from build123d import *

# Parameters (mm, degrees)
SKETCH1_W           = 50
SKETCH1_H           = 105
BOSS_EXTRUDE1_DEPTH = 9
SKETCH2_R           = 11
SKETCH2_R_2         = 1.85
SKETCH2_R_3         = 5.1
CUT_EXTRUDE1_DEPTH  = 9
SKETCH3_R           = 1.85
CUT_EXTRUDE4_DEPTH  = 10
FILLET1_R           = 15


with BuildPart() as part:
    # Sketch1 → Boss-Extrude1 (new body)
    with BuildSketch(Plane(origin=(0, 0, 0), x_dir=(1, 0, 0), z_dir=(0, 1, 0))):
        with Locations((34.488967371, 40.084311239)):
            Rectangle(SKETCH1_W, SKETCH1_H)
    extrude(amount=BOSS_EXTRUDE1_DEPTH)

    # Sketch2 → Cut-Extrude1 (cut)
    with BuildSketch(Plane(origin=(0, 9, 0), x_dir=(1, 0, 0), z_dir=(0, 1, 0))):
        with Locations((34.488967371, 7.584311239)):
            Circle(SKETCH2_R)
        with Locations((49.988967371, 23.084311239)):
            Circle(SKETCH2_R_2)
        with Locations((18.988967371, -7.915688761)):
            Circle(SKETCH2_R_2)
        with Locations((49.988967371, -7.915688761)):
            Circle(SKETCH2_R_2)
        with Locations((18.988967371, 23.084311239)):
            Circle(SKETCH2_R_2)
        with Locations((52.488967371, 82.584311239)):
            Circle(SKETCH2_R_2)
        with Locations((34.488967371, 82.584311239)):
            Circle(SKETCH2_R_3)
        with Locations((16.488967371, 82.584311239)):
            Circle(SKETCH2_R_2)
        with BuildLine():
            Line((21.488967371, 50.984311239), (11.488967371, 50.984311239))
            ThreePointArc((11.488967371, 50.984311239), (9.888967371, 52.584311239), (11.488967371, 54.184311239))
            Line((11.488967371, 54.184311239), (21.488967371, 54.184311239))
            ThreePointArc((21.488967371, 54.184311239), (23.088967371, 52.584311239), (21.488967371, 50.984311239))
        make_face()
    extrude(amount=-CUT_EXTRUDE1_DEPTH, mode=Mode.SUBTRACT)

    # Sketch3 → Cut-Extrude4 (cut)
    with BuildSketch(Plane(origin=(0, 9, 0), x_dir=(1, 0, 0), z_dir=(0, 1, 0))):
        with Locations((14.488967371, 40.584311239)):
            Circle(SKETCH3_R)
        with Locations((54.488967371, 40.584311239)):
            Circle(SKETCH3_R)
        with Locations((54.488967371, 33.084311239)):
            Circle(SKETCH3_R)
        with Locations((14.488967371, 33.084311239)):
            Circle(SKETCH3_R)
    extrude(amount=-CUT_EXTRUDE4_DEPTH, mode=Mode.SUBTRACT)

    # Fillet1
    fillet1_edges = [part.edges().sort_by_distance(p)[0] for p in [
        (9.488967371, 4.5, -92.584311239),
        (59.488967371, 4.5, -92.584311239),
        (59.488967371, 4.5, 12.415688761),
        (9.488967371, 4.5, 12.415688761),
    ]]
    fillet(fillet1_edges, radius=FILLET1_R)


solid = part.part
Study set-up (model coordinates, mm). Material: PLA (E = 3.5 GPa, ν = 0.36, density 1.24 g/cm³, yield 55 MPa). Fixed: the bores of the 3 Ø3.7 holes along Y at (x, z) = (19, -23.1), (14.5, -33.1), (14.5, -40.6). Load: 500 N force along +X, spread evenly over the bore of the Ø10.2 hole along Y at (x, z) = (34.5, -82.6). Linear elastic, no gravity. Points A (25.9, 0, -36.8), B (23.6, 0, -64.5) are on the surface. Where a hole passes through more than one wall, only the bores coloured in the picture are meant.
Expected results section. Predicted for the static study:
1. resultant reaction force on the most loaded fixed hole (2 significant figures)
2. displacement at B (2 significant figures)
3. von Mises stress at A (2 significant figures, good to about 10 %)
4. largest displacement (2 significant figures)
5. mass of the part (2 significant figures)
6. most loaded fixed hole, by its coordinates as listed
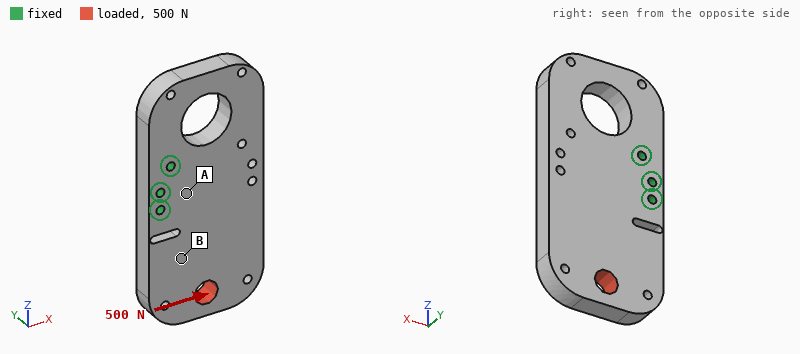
1.3 kN
0.21 mm
6.3 MPa
0.47 mm
50 g
(14.5, -40.6)
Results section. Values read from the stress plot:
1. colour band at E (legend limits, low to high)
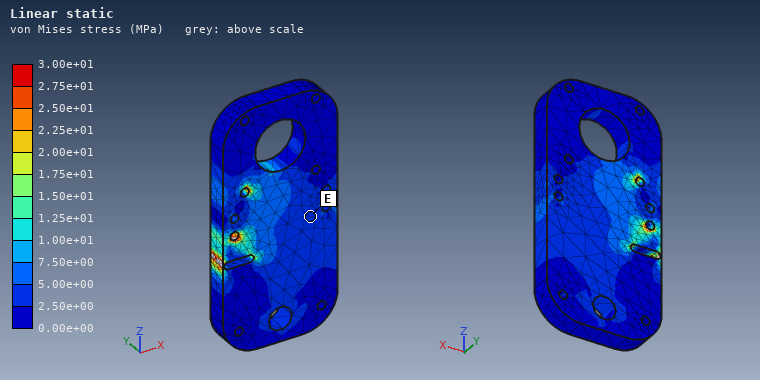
2.50e+00 to 5.00e+00 MPa
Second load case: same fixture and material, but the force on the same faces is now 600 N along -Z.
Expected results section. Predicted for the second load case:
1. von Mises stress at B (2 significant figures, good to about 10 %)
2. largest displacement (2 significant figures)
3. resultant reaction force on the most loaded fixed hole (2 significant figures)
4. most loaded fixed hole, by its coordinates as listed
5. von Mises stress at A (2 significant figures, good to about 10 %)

1.8 MPa
0.15 mm
640 N
(19, -23.1)
4.7 MPa
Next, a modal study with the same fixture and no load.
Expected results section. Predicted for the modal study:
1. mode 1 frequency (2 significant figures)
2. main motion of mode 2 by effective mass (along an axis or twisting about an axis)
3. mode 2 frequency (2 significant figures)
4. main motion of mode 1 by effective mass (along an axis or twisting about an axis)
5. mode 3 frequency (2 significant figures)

570 Hz
along Y
960 Hz
along Y
1300 Hz
